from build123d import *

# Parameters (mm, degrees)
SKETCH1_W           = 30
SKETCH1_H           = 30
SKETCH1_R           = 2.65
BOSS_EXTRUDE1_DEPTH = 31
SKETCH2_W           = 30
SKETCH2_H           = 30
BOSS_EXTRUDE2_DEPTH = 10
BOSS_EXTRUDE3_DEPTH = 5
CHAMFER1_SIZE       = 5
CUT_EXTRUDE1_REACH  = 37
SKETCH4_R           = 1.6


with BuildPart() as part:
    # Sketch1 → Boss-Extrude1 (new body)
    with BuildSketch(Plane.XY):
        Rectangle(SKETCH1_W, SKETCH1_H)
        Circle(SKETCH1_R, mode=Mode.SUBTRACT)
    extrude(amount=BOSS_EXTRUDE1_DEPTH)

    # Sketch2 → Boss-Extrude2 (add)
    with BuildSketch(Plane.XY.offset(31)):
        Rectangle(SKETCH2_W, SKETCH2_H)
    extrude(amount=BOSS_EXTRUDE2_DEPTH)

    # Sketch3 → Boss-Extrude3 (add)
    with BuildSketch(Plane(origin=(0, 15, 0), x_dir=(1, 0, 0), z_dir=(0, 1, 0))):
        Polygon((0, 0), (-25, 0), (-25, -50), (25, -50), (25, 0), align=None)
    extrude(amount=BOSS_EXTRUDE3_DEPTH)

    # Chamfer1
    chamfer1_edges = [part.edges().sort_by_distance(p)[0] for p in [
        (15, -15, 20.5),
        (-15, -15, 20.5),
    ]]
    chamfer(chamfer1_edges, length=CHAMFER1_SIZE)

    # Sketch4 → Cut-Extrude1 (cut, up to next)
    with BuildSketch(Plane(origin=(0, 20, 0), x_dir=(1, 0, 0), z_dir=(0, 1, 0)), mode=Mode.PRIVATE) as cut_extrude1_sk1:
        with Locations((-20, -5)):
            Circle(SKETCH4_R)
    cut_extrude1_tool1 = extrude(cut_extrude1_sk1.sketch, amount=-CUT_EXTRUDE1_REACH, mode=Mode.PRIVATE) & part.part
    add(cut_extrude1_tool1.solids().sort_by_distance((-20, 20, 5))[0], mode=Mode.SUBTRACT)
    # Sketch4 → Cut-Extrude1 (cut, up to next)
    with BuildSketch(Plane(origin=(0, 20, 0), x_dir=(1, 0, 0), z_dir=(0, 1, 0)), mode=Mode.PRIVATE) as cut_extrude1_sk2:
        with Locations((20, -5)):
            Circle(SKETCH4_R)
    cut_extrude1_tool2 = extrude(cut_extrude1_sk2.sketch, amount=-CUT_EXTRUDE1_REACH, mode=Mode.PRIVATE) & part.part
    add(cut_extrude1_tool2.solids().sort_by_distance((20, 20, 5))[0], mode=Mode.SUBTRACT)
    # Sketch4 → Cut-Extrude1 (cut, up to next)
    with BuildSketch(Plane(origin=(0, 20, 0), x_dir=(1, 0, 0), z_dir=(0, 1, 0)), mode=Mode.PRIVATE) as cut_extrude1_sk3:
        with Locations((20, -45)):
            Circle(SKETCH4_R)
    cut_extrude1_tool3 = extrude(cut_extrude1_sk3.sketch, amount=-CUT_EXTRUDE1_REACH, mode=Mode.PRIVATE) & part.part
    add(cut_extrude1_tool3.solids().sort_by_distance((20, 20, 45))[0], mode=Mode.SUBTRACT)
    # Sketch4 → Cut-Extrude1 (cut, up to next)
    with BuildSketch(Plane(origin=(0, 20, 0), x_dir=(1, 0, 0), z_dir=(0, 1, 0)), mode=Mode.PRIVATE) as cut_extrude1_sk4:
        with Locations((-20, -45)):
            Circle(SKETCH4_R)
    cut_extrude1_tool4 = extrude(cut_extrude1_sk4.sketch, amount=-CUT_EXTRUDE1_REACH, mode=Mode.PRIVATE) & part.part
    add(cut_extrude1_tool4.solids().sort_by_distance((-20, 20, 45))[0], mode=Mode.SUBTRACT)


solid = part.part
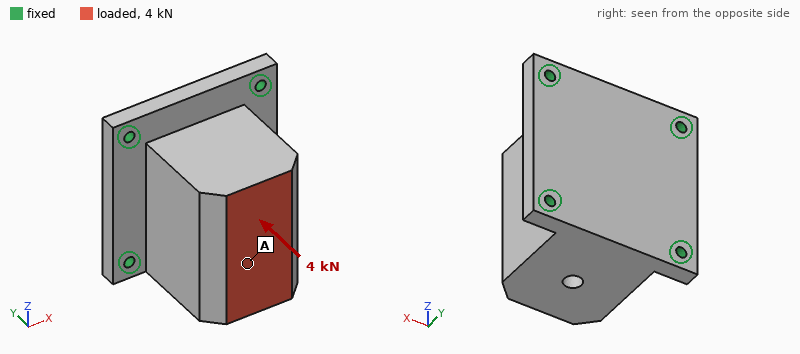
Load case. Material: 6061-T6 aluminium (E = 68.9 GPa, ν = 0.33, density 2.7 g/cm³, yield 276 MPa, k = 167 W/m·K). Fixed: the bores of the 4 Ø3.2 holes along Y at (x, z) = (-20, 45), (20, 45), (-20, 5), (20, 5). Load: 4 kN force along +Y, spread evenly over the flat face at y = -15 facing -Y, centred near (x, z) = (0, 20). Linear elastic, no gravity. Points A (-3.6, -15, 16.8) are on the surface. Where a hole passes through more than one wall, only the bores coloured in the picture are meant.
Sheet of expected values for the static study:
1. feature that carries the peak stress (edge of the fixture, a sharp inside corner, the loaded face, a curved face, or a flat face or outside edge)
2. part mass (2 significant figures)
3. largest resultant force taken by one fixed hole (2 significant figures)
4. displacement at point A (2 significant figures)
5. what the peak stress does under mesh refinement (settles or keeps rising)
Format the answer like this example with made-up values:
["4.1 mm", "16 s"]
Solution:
["edge of the fixture", "130 g", "1.3 kN", "14 µm", "keeps rising"]
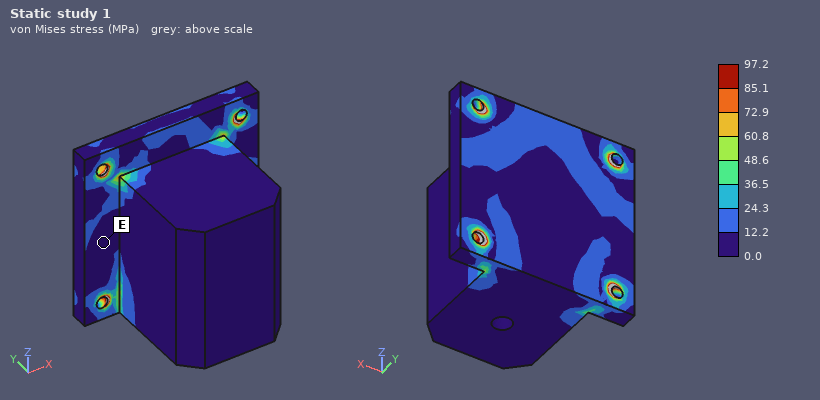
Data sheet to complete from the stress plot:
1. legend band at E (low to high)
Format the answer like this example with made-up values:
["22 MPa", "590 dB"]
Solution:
["0.0 to 12.2 MPa"]
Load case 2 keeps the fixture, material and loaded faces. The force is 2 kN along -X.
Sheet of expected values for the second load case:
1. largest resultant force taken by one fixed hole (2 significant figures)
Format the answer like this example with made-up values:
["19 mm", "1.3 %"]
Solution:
["1.4 kN"]
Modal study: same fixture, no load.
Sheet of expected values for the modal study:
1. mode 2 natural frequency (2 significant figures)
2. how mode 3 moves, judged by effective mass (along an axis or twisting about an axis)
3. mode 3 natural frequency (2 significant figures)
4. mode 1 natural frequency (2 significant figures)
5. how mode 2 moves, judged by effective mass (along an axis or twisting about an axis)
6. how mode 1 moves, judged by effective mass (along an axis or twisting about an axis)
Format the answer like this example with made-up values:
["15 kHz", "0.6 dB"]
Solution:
["7000 Hz", "along Y", "8400 Hz", "6500 Hz", "along X", "along Z"]
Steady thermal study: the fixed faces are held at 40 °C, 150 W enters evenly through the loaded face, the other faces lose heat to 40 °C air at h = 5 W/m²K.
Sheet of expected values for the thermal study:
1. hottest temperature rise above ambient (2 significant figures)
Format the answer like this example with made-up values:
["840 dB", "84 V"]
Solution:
["55 K"]
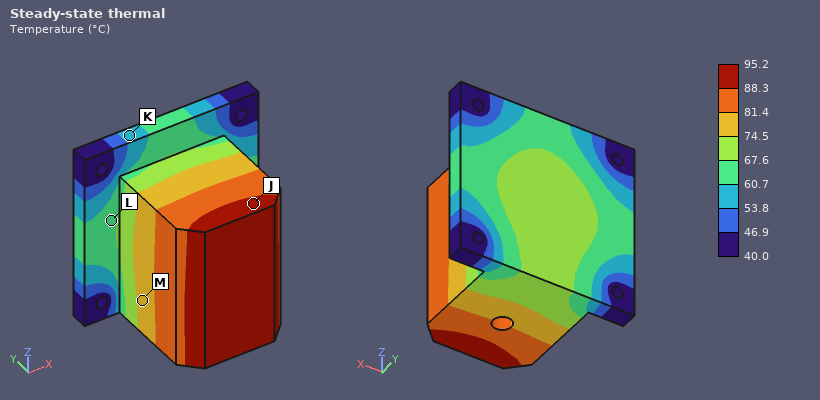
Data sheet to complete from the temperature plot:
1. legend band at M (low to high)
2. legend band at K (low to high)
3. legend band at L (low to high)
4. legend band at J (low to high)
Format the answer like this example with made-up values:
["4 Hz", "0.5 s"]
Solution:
["74.5 to 81.4 °C", "53.8 to 60.7 °C", "60.7 to 67.6 °C", "88.3 to 95.2 °C"]
